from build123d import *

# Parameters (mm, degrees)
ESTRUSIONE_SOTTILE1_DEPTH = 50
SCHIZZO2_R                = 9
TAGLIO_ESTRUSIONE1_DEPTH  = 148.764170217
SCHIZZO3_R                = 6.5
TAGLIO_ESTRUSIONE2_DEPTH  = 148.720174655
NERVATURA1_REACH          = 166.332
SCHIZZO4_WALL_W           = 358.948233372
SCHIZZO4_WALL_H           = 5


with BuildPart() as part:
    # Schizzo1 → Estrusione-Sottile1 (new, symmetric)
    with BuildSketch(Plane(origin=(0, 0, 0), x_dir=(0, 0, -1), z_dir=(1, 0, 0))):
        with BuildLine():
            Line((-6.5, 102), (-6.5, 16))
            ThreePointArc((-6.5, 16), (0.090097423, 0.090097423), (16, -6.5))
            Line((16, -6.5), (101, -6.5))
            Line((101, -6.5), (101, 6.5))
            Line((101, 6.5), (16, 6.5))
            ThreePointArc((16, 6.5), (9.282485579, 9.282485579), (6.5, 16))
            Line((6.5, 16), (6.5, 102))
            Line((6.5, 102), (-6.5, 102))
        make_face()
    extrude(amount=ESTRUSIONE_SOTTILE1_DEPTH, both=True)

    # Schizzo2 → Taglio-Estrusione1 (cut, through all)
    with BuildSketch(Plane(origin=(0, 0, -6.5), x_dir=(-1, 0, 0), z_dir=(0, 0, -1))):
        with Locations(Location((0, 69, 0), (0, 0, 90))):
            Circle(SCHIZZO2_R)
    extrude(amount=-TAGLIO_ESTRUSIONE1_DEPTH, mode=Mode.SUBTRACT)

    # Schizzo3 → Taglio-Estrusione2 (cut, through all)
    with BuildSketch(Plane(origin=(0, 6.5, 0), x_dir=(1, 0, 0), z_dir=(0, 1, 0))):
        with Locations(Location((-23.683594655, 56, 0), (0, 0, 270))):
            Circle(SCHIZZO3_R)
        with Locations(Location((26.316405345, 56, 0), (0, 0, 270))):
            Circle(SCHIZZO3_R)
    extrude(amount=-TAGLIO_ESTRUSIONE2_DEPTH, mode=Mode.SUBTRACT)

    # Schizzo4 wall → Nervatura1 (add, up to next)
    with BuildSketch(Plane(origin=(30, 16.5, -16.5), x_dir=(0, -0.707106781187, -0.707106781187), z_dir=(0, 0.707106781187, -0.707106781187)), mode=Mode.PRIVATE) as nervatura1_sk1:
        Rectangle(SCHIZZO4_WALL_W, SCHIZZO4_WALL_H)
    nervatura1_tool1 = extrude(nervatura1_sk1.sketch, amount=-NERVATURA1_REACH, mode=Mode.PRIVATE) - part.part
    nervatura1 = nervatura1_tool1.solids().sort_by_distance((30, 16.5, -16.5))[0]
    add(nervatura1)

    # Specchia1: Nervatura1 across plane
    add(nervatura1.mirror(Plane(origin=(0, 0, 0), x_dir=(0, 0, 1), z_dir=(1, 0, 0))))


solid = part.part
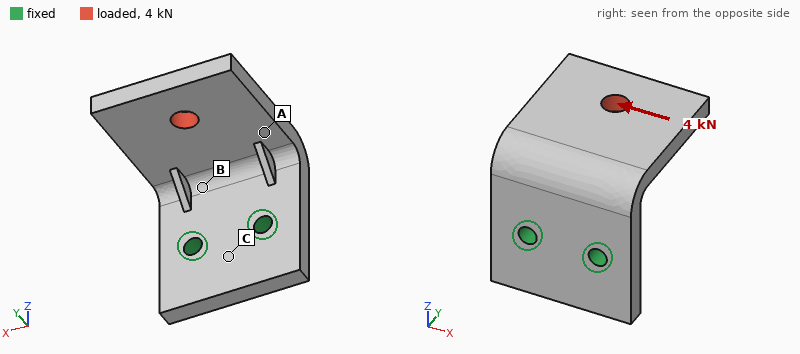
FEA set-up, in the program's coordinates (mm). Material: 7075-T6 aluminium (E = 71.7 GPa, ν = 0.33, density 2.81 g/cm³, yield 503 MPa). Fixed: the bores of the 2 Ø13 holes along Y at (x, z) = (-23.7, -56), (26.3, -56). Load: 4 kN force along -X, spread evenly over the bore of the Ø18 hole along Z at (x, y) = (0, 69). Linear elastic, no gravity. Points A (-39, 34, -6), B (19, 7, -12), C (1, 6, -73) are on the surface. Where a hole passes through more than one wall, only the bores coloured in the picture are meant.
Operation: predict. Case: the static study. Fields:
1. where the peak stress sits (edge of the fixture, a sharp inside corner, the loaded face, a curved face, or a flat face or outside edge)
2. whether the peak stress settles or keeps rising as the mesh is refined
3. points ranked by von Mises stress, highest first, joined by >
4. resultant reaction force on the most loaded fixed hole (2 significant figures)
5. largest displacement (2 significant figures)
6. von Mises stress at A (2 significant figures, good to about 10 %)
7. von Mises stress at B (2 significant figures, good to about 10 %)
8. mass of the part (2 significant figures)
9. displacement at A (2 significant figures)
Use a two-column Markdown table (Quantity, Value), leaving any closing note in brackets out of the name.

| Quantity | Value |
|---|---|
| where the peak stress sits | edge of the fixture |
| whether the peak stress settles or keeps rising as the mesh is refined | keeps rising |
| points ranked by von Mises stress, highest first, joined by > | B > A > C |
| resultant reaction force on the most loaded fixed hole | 6.0 kN |
| largest displacement | 0.44 mm |
| von Mises stress at A | 26 MPa |
| von Mises stress at B | 58 MPa |
| mass of the part | 700 g |
| displacement at A | 0.20 mm |
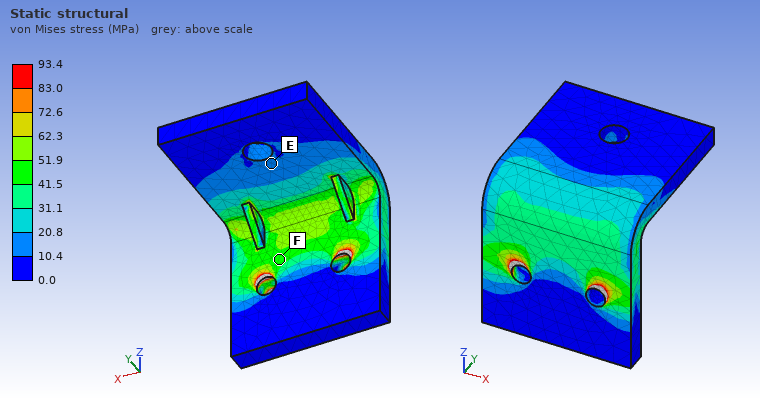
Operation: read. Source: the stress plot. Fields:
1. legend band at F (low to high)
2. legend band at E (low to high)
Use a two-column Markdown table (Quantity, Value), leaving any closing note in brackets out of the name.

| Quantity | Value |
|---|---|
| legend band at F | 41.5 to 51.9 MPa |
| legend band at E | 10.4 to 20.8 MPa |
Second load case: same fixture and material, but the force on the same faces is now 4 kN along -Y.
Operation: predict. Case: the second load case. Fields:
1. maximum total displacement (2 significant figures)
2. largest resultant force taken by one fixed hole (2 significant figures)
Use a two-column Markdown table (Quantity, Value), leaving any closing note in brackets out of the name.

| Quantity | Value |
|---|---|
| maximum total displacement | 0.47 mm |
| largest resultant force taken by one fixed hole | 2.1 kN |
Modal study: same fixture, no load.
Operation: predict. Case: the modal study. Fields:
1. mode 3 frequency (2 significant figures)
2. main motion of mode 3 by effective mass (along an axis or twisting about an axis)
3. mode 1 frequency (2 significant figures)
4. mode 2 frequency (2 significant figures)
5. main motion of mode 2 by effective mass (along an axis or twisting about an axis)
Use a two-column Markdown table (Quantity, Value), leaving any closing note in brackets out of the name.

| Quantity | Value |
|---|---|
| mode 3 frequency | 2100 Hz |
| main motion of mode 3 by effective mass | along Y |
| mode 1 frequency | 620 Hz |
| mode 2 frequency | 1100 Hz |
| main motion of mode 2 by effective mass | along X |
